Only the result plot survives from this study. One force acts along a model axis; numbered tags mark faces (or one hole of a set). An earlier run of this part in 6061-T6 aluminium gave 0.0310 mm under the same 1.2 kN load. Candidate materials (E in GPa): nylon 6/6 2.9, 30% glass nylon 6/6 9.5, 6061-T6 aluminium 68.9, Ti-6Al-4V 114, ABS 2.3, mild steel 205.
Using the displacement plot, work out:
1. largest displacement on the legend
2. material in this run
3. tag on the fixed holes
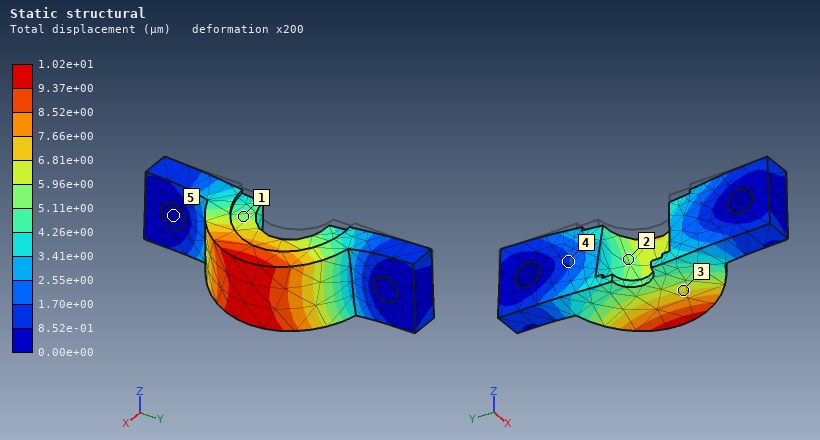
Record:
1.02e+01 µm
mild steel
5
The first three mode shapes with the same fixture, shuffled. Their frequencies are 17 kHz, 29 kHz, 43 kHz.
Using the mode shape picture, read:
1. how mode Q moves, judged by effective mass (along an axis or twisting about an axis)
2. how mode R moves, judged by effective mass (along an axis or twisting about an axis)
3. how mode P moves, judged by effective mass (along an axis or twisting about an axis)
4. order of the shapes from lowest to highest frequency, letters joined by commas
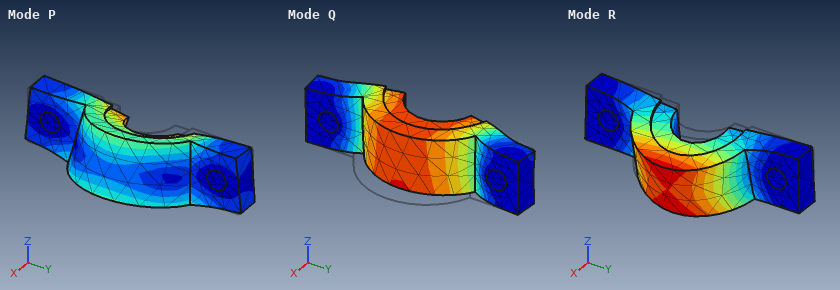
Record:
along X
along Z
along Z
R, Q, P
